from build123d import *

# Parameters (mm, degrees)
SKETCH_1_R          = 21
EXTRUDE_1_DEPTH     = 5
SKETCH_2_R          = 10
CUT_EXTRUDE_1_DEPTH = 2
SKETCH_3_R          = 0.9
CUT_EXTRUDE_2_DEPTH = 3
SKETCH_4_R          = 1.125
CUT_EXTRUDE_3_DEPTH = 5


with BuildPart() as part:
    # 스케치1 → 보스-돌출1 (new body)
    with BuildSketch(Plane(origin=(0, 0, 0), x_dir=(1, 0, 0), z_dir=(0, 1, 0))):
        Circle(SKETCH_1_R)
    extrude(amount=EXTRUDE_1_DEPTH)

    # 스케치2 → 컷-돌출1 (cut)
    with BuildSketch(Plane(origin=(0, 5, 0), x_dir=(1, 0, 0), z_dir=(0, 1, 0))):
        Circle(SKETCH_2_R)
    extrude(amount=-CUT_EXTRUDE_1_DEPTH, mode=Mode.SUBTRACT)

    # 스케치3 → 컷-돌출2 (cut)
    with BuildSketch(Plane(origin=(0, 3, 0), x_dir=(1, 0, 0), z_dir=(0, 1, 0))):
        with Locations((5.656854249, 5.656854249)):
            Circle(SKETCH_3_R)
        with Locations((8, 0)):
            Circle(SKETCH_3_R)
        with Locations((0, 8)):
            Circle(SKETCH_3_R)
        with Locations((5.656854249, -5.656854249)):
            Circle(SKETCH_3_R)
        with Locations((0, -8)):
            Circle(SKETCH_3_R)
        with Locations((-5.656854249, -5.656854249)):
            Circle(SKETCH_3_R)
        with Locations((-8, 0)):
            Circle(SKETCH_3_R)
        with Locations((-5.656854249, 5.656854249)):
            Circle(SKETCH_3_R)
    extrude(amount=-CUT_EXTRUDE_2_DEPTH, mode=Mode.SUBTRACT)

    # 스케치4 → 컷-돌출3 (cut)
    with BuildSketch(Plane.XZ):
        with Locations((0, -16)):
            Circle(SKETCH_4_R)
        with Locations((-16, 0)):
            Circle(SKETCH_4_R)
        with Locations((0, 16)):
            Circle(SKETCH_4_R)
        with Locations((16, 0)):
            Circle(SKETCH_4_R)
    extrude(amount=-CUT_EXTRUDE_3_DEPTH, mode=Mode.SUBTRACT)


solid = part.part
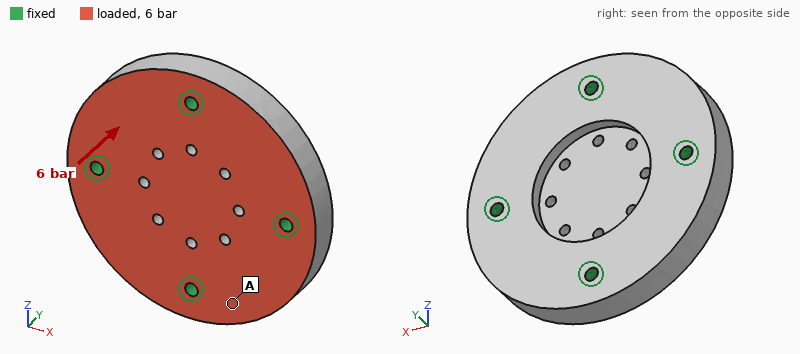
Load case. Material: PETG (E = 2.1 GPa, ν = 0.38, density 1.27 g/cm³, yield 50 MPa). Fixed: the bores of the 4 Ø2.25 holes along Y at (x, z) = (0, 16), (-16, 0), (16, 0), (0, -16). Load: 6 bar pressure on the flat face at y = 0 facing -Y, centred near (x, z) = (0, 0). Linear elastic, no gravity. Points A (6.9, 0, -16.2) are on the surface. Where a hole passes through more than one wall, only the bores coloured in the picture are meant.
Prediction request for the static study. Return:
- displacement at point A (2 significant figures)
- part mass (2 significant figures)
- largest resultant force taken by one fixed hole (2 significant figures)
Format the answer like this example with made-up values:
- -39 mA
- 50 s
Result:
- 33 µm
- 7.8 g
- 200 N
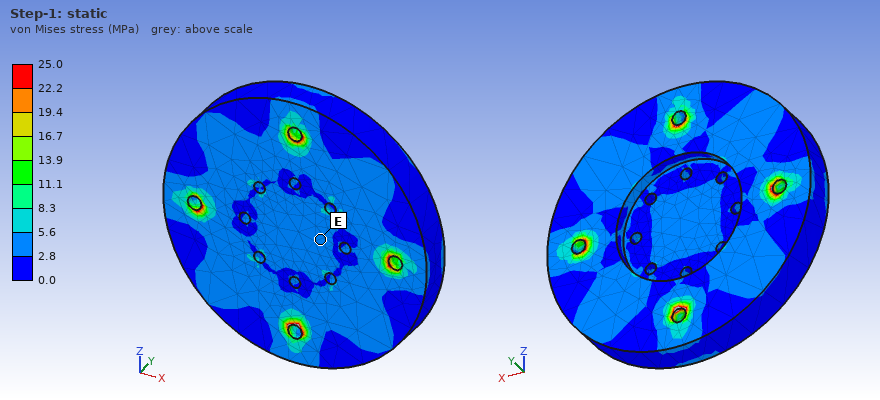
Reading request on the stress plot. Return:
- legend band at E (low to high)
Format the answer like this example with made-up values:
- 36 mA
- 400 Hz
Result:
- 2.8 to 5.6 MPa
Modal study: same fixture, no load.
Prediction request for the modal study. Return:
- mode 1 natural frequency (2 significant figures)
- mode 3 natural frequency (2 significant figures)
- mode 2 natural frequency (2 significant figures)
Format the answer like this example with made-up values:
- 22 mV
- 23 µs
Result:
- 6500 Hz
- 7100 Hz
- 7100 Hz
